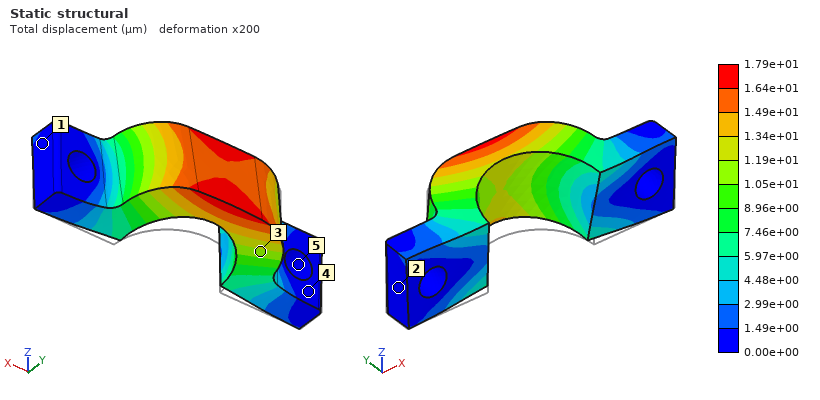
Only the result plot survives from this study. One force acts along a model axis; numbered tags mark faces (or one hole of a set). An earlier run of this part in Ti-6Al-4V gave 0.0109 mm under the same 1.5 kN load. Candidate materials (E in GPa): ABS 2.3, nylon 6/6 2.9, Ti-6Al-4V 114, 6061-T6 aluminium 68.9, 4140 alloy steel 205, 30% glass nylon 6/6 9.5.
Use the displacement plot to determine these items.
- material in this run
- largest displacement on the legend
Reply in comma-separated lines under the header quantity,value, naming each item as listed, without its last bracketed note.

quantity,value
material in this run,6061-T6 aluminium
largest displacement on the legend,1.79e+01 µm
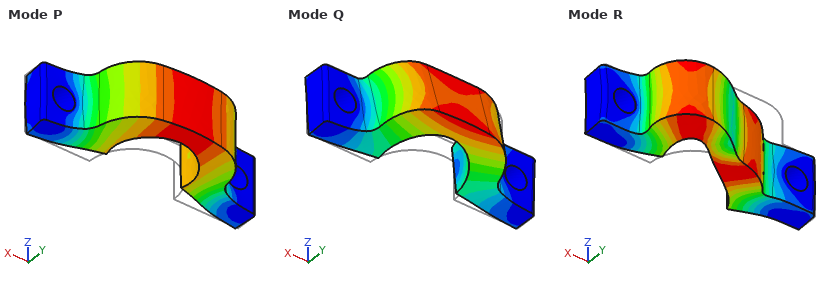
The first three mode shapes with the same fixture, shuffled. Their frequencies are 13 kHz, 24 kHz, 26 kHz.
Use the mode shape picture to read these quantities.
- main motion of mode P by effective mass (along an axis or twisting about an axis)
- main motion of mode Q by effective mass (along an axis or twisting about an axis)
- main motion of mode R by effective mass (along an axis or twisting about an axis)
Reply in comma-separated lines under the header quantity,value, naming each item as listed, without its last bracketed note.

quantity,value
main motion of mode P by effective mass,along Y
main motion of mode Q by effective mass,along Z
main motion of mode R by effective mass,along X
